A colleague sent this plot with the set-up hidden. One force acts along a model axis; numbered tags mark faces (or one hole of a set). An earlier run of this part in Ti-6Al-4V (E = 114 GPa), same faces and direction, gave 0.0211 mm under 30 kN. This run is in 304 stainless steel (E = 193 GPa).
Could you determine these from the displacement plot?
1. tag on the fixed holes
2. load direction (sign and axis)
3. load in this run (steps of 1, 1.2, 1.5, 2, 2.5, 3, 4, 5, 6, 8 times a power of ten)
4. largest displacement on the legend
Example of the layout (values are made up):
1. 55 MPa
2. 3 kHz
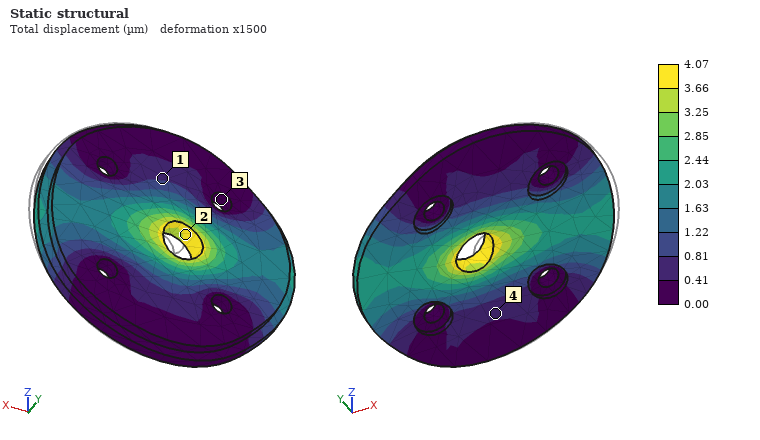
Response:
1. 3
2. -X
3. 10 kN
4. 4.07 µm
